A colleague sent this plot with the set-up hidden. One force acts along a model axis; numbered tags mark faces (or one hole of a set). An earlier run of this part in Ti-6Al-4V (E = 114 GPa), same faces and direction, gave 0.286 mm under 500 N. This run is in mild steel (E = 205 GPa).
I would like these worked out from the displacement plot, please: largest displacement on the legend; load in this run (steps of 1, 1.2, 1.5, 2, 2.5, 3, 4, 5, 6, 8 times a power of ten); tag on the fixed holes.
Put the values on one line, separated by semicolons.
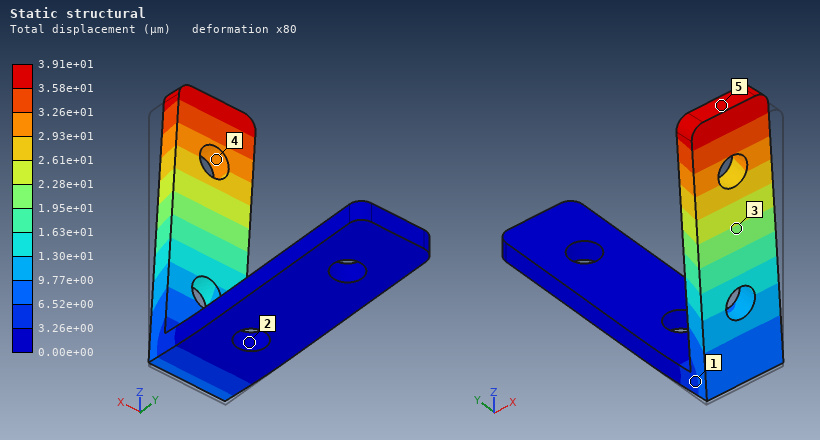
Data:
3.91e+01 µm; 120 N; 2
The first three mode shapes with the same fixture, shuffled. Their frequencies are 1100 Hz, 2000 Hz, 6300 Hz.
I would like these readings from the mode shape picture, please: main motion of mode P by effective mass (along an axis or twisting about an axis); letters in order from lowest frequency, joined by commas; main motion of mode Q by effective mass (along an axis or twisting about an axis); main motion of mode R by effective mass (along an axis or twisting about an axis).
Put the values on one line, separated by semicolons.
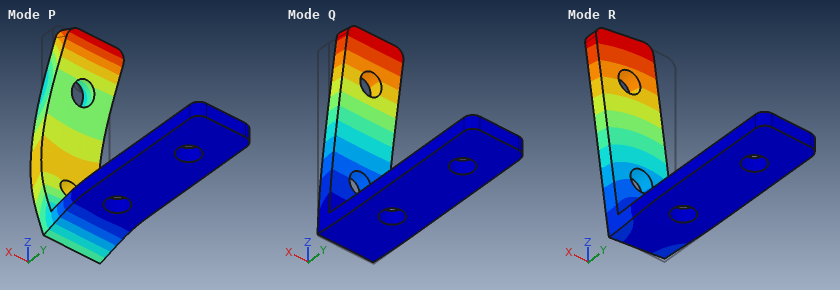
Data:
along Z; Q, R, P; along Y; along X
